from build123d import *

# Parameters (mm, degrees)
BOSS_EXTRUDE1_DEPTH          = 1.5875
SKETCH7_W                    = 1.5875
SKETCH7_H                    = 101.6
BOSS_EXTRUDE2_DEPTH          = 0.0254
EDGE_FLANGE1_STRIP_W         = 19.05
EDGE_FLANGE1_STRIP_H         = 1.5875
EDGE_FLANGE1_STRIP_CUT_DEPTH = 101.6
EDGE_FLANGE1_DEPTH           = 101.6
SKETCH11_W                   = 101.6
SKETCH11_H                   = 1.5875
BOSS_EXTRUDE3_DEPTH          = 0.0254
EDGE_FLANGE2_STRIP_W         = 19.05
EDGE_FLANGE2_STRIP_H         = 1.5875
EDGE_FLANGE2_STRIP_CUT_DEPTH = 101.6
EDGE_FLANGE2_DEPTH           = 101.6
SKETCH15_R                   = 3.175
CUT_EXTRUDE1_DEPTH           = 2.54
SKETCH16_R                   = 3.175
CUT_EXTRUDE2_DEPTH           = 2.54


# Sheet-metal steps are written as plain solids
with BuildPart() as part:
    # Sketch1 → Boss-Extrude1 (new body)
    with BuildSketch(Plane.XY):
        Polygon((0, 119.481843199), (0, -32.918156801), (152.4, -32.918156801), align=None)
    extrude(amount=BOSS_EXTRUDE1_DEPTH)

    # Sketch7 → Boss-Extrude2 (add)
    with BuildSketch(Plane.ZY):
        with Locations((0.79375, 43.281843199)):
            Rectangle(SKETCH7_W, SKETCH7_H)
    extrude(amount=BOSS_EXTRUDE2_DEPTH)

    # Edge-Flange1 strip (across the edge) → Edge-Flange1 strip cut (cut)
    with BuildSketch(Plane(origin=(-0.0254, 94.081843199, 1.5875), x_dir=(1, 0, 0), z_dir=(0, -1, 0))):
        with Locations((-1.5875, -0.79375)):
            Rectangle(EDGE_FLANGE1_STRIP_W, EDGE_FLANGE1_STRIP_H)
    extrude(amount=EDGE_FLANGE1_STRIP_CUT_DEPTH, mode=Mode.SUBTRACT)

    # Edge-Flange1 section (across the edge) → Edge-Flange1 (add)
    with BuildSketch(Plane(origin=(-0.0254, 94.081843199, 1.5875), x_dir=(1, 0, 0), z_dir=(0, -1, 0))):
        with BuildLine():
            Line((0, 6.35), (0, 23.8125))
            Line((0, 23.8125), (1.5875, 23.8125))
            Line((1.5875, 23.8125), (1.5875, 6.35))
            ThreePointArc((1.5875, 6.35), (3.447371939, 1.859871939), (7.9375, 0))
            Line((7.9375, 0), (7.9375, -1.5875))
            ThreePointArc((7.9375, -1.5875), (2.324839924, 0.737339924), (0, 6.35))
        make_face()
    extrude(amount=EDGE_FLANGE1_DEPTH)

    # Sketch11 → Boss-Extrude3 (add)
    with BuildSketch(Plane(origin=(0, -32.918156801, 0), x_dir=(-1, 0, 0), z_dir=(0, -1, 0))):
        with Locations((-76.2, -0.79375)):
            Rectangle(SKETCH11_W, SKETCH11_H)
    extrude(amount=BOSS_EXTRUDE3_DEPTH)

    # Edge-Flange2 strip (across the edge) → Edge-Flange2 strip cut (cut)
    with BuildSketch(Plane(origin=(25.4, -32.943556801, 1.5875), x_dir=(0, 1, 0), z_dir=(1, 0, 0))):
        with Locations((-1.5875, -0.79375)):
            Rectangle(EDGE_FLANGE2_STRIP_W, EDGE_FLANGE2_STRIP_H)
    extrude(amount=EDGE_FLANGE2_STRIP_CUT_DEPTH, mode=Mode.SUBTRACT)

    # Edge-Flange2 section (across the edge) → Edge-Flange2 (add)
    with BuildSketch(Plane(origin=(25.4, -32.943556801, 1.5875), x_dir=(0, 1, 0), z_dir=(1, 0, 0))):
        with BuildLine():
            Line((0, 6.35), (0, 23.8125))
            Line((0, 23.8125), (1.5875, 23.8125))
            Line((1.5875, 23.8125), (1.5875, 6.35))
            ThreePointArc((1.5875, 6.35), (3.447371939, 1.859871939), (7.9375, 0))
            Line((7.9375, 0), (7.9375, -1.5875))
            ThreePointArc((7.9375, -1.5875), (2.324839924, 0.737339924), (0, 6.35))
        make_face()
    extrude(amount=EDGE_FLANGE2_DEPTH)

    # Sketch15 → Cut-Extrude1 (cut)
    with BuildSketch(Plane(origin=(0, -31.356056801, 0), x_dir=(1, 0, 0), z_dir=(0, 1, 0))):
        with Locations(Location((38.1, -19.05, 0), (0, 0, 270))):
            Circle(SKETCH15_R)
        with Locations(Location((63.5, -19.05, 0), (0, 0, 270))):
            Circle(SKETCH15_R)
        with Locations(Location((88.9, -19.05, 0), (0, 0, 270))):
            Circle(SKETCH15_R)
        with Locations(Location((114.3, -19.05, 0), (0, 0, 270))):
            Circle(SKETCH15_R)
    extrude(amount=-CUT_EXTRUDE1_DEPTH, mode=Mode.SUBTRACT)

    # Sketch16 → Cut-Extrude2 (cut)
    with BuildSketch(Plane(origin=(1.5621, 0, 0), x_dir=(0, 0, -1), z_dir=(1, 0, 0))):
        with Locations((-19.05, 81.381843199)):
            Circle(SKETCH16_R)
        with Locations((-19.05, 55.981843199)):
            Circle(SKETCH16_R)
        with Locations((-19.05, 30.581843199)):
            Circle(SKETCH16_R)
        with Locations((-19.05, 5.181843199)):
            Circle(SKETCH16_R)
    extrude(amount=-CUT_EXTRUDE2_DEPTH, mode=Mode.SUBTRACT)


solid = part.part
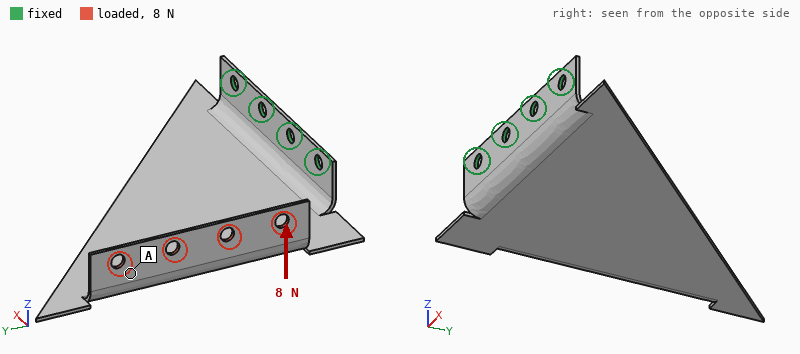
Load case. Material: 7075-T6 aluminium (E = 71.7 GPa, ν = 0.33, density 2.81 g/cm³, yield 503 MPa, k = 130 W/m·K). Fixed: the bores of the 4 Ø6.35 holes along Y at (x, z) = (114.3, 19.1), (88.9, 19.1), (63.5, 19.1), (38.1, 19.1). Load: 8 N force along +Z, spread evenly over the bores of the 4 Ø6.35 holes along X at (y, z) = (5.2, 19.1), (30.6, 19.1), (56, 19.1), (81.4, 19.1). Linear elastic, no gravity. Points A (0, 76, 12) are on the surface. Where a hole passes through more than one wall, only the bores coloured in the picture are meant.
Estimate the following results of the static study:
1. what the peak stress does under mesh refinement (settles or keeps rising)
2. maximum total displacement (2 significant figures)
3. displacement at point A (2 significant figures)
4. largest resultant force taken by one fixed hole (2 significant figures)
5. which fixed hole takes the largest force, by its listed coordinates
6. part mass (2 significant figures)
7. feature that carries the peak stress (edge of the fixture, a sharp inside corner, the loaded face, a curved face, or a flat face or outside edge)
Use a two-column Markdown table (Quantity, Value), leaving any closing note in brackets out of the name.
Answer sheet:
| Quantity | Value |
|---|---|
| what the peak stress does under mesh refinement | keeps rising |
| maximum total displacement | 2.4 mm |
| displacement at point A | 1.7 mm |
| largest resultant force taken by one fixed hole | 11 N |
| which fixed hole takes the largest force, by its listed coordinates | (38.1, 19.1) |
| part mass | 70 g |
| feature that carries the peak stress | a sharp inside corner |
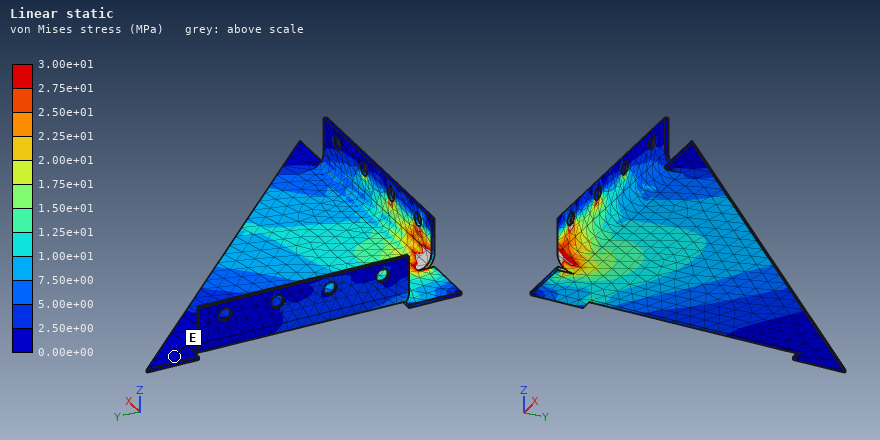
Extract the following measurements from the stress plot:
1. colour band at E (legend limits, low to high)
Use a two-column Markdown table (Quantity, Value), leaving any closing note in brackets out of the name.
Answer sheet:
| Quantity | Value |
|---|---|
| colour band at E | 0.00e+00 to 2.50e+00 MPa |
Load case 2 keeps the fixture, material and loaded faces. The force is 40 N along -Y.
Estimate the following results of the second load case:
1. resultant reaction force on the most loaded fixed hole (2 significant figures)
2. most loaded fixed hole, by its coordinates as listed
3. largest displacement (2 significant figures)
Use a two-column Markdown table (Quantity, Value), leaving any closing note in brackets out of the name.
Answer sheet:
| Quantity | Value |
|---|---|
| resultant reaction force on the most loaded fixed hole | 48 N |
| most loaded fixed hole, by its coordinates as listed | (38.1, 19.1) |
| largest displacement | 2.4 mm |
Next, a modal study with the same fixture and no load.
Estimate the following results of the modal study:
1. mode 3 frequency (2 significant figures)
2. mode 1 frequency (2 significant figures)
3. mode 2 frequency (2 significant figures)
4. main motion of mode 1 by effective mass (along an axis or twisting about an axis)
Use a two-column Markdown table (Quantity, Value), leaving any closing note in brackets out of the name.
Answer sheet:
| Quantity | Value |
|---|---|
| mode 3 frequency | 390 Hz |
| mode 1 frequency | 70 Hz |
| mode 2 frequency | 280 Hz |
| main motion of mode 1 by effective mass | along Z |
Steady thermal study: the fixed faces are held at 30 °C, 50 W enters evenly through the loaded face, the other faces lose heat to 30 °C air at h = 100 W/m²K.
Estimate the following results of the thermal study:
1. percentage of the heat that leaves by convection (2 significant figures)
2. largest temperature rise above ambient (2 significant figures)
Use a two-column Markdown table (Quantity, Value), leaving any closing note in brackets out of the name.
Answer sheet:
| Quantity | Value |
|---|---|
| percentage of the heat that leaves by convection | 97 % |
| largest temperature rise above ambient | 74 K |
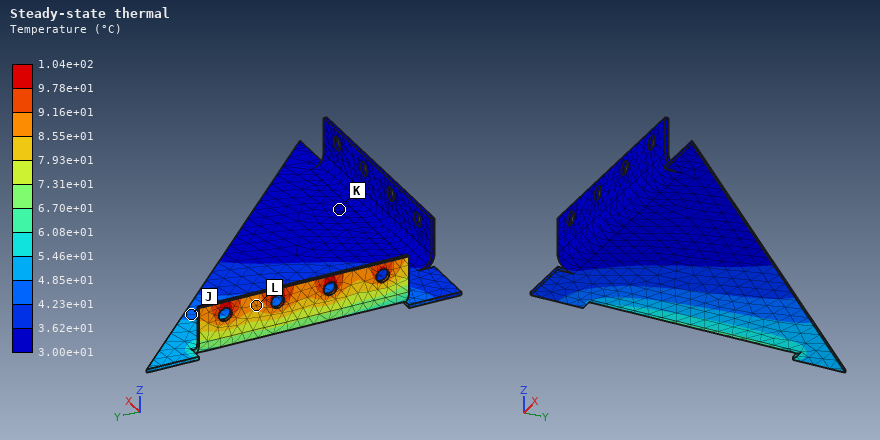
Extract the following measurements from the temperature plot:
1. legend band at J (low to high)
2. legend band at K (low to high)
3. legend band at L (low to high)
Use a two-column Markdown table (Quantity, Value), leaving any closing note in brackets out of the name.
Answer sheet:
| Quantity | Value |
|---|---|
| legend band at J | 4.23e+01 to 4.85e+01 °C |
| legend band at K | 3.00e+01 to 3.62e+01 °C |
| legend band at L | 8.55e+01 to 9.16e+01 °C |
